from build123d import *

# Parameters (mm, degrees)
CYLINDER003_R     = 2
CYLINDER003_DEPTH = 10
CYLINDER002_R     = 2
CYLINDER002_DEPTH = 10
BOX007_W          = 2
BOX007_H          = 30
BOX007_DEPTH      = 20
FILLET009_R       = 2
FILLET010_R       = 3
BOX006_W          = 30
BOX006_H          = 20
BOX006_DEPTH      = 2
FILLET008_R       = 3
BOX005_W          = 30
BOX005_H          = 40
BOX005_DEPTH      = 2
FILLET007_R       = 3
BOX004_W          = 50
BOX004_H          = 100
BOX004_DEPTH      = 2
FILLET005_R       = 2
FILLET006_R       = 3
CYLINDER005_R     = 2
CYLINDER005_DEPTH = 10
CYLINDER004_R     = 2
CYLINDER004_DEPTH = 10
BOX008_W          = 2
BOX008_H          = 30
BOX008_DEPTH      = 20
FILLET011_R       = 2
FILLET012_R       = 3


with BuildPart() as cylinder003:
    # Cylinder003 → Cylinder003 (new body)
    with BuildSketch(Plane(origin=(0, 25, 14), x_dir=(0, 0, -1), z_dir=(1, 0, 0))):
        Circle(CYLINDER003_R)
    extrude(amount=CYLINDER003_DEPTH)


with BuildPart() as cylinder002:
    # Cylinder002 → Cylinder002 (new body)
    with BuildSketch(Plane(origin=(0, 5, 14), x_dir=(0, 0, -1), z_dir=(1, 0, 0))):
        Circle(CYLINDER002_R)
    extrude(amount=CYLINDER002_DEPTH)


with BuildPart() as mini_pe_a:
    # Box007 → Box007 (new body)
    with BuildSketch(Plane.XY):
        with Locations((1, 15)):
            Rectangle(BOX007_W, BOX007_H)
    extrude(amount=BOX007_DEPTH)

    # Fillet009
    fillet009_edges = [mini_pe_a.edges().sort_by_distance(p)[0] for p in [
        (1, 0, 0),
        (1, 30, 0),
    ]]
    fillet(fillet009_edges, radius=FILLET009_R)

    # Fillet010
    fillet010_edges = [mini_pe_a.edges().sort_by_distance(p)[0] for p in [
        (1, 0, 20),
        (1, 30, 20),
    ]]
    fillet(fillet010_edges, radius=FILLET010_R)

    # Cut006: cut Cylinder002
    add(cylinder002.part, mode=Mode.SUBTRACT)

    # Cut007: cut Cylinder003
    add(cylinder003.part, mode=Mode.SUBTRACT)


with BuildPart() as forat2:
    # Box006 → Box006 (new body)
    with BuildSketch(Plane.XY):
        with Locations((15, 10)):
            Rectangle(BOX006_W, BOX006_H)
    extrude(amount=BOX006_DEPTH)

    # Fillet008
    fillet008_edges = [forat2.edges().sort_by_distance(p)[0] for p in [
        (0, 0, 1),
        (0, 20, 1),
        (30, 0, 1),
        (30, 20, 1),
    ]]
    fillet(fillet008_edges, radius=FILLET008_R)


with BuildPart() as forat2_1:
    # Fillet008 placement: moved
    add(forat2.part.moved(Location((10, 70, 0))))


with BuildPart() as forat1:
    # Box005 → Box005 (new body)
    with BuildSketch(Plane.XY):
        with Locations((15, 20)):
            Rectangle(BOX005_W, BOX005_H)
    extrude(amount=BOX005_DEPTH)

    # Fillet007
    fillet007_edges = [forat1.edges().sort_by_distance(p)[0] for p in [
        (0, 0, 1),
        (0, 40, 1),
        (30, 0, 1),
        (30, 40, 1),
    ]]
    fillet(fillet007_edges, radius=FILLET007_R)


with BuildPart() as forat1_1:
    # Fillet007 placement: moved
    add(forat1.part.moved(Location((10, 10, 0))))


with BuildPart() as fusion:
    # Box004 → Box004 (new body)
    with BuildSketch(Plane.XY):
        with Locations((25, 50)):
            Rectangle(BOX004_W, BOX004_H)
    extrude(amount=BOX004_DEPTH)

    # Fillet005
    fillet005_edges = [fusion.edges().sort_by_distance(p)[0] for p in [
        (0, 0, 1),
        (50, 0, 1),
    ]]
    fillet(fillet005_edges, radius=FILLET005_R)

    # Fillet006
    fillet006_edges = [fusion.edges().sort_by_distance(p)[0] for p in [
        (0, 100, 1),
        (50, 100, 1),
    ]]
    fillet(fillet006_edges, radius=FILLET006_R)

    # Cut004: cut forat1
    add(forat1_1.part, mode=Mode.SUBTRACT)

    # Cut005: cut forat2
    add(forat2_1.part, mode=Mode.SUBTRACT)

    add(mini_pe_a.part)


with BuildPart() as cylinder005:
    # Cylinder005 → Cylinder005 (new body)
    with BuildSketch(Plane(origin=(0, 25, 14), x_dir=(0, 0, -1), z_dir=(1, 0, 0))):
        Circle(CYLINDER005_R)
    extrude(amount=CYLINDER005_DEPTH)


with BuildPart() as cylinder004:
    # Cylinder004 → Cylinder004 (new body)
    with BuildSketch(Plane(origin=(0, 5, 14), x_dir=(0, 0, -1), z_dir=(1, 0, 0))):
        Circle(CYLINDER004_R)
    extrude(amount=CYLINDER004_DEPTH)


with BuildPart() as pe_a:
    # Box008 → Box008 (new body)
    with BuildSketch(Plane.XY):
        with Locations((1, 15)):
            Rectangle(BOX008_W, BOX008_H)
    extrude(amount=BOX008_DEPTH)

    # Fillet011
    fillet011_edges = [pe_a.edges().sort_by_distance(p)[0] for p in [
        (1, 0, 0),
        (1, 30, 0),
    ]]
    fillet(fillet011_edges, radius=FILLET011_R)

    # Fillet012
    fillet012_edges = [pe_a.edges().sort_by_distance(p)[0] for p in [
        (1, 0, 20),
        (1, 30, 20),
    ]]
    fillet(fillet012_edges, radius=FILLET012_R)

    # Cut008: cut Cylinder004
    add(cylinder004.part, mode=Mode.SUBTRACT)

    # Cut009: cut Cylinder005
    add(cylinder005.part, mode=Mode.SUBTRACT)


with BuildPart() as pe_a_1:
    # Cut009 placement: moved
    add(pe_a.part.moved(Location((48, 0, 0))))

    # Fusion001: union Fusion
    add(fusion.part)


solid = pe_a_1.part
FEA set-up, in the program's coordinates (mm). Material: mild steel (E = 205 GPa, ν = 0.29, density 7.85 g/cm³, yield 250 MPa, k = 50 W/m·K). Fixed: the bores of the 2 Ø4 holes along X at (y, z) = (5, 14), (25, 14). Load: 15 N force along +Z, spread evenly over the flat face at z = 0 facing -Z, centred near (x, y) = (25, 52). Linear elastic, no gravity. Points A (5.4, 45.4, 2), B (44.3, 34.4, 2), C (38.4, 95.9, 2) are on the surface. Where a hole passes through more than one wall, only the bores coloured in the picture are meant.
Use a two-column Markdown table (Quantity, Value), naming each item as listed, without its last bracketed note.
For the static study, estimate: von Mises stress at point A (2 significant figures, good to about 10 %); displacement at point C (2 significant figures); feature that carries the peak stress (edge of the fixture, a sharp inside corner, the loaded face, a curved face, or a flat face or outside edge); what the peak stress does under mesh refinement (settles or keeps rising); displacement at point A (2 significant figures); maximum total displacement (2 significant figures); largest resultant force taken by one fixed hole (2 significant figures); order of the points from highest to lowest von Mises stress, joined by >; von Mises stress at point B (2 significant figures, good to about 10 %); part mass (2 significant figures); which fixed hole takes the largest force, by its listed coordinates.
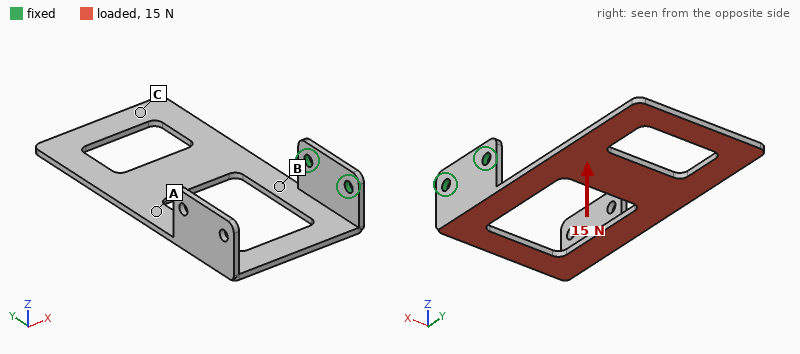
| Quantity | Value |
|---|---|
| von Mises stress at point A | 15 MPa |
| displacement at point C | 0.31 mm |
| feature that carries the peak stress | a sharp inside corner |
| what the peak stress does under mesh refinement | keeps rising |
| displacement at point A | 0.21 mm |
| maximum total displacement | 0.48 mm |
| largest resultant force taken by one fixed hole | 34 N |
| order of the points from highest to lowest von Mises stress, joined by > | B > A > C |
| von Mises stress at point B | 44 MPa |
| part mass | 66 g |
| which fixed hole takes the largest force, by its listed coordinates | (25, 14) |
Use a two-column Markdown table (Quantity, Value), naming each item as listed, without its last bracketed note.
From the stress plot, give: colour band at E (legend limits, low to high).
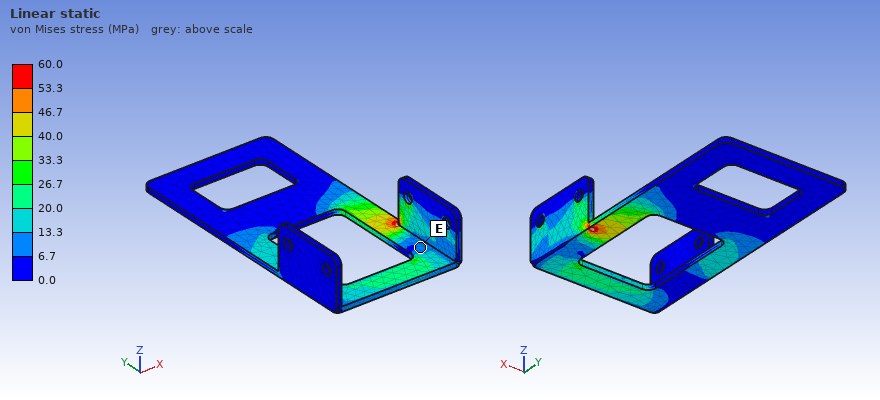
| Quantity | Value |
|---|---|
| colour band at E | 6.7 to 13.3 MPa |
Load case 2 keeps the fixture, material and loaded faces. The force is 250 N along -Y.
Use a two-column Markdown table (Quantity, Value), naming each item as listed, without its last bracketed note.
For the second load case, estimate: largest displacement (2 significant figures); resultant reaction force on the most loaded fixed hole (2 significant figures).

| Quantity | Value |
|---|---|
| largest displacement | 0.40 mm |
| resultant reaction force on the most loaded fixed hole | 340 N |
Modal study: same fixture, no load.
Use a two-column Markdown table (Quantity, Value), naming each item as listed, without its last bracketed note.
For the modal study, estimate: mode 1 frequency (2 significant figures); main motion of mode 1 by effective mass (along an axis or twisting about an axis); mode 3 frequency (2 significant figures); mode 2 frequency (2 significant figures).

| Quantity | Value |
|---|---|
| mode 1 frequency | 160 Hz |
| main motion of mode 1 by effective mass | along Z |
| mode 3 frequency | 450 Hz |
| mode 2 frequency | 300 Hz |
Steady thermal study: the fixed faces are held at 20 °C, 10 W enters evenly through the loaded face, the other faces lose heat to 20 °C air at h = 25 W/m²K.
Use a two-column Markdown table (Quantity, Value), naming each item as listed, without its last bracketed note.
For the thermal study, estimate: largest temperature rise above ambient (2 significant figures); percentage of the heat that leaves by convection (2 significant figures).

| Quantity | Value |
|---|---|
| largest temperature rise above ambient | 72 K |
| percentage of the heat that leaves by convection | 68 % |
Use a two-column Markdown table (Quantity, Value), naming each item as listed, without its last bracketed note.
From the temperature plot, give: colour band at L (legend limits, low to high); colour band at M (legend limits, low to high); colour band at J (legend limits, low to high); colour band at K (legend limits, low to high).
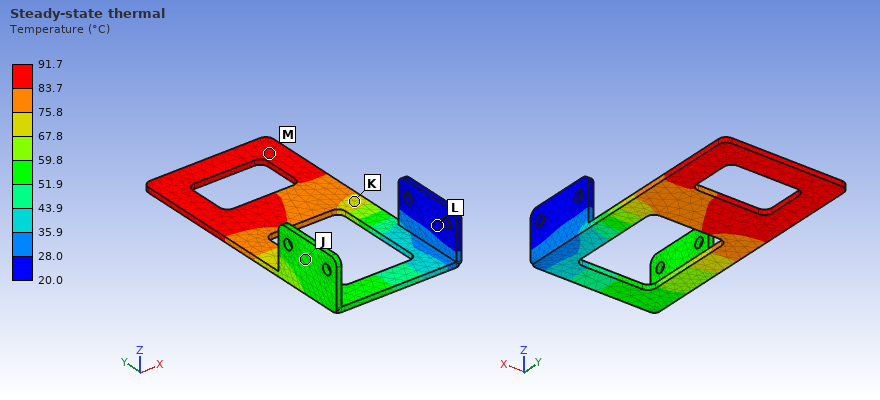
| Quantity | Value |
|---|---|
| colour band at L | 20.0 to 28.0 °C |
| colour band at M | 83.7 to 91.7 °C |
| colour band at J | 51.9 to 59.8 °C |
| colour band at K | 67.8 to 75.8 °C |
